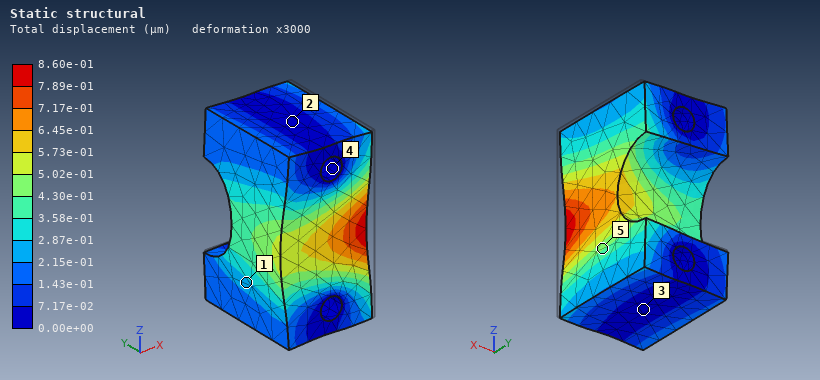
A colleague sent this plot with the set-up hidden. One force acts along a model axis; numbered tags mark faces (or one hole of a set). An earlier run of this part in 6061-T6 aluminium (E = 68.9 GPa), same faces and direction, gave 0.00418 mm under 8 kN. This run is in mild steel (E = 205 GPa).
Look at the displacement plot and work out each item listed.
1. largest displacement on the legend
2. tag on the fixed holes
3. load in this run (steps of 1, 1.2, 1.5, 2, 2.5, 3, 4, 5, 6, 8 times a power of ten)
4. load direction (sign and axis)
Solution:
8.60e-01 µm
4
5 kN
-X
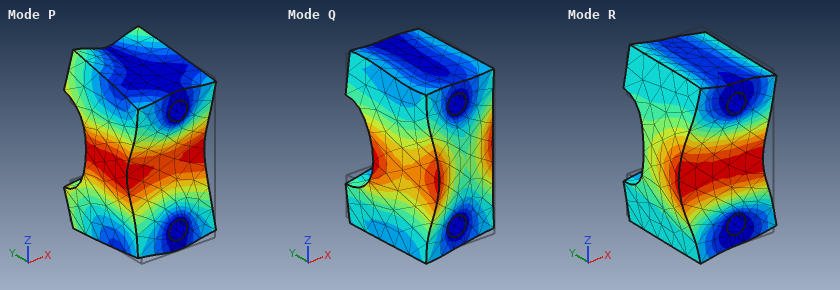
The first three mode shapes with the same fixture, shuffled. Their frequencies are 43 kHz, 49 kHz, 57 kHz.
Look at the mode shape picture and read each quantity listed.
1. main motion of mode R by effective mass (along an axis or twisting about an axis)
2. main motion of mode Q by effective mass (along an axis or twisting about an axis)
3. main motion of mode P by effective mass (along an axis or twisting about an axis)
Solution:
along X
twisting about Z
along Y
